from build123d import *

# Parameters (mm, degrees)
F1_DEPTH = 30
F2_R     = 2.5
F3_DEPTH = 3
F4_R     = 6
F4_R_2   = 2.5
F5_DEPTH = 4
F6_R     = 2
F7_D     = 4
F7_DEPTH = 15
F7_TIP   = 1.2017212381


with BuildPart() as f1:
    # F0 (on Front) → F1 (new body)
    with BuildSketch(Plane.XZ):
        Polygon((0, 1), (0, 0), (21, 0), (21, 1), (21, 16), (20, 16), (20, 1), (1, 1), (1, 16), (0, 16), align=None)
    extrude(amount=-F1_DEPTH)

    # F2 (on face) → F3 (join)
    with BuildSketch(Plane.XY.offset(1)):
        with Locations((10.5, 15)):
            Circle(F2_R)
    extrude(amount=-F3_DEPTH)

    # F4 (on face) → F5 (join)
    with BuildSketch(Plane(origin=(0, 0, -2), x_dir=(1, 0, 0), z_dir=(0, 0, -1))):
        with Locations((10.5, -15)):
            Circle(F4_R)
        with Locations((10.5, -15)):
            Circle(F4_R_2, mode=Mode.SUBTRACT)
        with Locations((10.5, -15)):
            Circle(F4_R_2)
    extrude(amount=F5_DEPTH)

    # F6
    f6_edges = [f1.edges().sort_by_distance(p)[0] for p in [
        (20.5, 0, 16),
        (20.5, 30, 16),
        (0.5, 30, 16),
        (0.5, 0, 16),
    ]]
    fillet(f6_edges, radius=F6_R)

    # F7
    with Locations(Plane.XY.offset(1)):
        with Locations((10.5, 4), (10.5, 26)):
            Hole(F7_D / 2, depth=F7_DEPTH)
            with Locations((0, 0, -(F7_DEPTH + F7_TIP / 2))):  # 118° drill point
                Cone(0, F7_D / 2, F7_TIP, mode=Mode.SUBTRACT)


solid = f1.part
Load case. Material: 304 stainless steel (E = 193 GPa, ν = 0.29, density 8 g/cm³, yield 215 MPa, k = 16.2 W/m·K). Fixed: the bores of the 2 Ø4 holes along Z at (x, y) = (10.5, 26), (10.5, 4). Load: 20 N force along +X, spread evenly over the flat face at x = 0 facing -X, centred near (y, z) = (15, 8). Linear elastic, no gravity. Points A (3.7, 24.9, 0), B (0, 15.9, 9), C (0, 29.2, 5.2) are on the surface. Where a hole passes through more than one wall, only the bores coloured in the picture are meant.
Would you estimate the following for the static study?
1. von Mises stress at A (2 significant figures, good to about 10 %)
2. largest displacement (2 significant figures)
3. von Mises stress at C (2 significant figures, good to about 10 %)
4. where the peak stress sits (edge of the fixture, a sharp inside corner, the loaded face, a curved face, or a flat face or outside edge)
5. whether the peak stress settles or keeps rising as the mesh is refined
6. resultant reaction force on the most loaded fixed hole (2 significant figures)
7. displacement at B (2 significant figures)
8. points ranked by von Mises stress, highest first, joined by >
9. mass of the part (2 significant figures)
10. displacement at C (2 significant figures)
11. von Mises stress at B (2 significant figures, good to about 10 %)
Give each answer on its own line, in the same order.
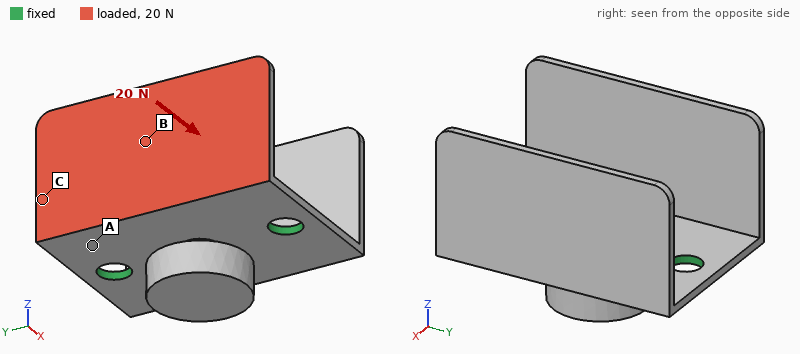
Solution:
26 MPa
58 µm
14 MPa
edge of the fixture
keeps rising
10 N
32 µm
A > C > B
16 g
20 µm
5.4 MPa
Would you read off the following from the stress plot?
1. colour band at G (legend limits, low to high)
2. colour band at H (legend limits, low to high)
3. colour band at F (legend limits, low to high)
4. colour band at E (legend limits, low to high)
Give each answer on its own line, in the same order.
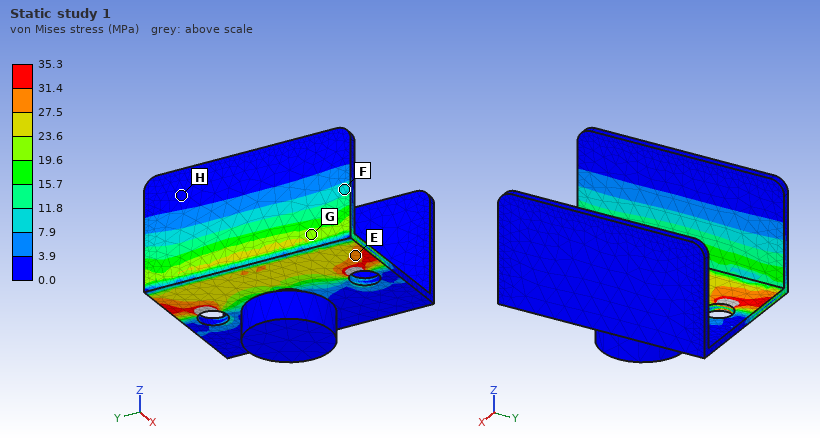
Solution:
19.6 to 23.6 MPa
0.0 to 3.9 MPa
7.9 to 11.8 MPa
27.5 to 31.4 MPa
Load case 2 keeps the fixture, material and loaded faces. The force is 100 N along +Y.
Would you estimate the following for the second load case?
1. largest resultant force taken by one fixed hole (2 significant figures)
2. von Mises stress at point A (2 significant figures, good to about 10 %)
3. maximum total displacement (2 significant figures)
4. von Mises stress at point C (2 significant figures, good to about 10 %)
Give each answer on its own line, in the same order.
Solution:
73 N
33 MPa
43 µm
23 MPa
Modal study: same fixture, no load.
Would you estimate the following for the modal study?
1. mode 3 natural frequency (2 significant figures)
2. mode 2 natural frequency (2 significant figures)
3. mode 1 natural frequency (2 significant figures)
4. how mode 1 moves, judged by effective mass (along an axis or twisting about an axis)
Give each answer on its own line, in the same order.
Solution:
3400 Hz
1800 Hz
1700 Hz
along X
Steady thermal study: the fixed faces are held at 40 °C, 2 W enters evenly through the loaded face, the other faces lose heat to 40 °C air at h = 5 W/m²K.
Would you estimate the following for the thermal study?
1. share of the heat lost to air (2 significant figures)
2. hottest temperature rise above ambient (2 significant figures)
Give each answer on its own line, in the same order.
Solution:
13 %
66 K
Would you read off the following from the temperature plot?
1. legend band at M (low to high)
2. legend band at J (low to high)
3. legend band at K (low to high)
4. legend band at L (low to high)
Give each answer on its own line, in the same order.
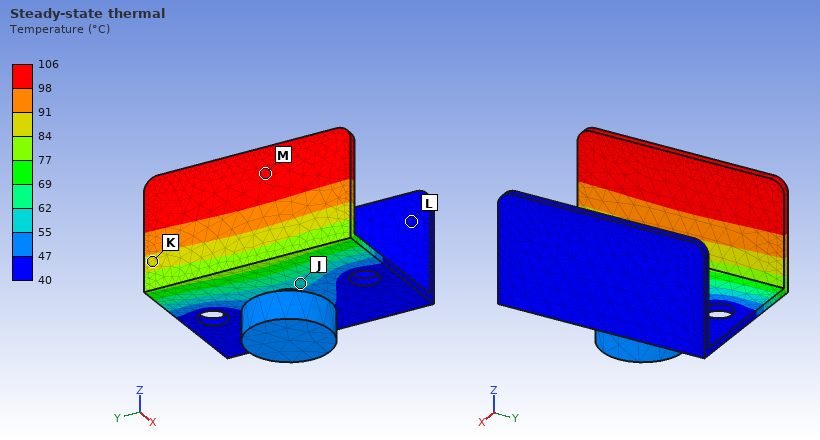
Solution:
98 to 106 °C
55 to 62 °C
84 to 91 °C
40 to 47 °C
